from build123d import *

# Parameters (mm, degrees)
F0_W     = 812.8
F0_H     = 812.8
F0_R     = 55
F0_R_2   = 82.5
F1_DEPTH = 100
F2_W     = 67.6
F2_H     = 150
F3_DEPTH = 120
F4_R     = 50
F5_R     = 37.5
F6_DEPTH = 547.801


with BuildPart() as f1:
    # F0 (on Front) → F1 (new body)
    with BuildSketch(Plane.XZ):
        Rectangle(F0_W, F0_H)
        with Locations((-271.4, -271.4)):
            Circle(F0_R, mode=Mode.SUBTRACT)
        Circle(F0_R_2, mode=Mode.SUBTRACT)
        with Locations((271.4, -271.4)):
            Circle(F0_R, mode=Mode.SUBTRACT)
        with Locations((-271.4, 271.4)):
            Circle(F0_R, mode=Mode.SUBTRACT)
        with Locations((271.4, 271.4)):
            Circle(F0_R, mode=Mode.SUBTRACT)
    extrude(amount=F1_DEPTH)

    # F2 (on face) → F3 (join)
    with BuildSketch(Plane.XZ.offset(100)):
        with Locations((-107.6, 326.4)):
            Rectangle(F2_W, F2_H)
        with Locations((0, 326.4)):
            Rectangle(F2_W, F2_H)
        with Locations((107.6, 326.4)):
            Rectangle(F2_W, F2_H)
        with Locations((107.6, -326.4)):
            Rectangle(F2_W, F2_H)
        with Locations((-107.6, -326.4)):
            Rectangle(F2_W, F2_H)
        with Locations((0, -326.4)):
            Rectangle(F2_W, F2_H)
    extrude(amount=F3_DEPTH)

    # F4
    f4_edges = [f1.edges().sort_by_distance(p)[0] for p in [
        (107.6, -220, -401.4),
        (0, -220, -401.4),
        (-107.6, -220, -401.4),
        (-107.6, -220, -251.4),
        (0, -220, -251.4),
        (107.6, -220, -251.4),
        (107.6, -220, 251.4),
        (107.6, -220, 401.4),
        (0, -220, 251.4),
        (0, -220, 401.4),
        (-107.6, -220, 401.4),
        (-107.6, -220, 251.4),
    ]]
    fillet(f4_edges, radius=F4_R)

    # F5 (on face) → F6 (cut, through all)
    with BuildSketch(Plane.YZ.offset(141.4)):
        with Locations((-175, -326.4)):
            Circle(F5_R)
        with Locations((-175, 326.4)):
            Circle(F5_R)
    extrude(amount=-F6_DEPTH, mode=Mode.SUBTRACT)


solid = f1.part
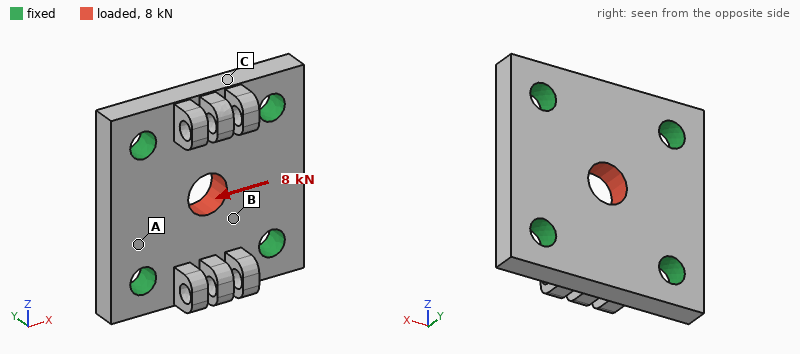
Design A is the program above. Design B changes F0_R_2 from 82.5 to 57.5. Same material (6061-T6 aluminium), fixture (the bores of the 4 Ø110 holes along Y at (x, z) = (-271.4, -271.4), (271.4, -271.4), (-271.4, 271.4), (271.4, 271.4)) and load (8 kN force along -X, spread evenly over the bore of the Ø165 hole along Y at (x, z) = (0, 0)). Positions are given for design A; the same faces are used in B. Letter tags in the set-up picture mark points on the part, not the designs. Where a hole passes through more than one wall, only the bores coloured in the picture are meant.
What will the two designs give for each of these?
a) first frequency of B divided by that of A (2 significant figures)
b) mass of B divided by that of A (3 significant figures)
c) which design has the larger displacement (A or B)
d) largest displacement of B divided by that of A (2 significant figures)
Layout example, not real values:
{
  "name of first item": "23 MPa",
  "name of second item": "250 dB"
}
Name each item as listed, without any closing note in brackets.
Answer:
{
  "first frequency of B divided by that of A": "0.98",
  "mass of B divided by that of A": "1.02",
  "which design has the larger displacement": "B",
  "largest displacement of B divided by that of A": "1.2"
}
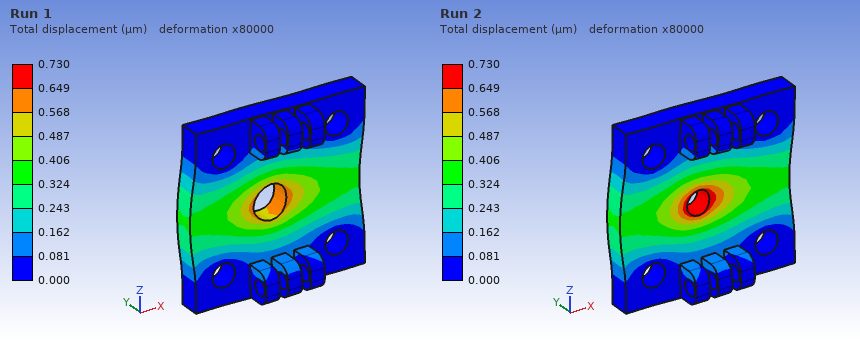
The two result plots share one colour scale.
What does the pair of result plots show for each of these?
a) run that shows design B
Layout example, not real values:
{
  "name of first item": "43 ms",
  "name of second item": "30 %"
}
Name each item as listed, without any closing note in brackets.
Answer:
{
  "run that shows design B": "Run 2"
}
